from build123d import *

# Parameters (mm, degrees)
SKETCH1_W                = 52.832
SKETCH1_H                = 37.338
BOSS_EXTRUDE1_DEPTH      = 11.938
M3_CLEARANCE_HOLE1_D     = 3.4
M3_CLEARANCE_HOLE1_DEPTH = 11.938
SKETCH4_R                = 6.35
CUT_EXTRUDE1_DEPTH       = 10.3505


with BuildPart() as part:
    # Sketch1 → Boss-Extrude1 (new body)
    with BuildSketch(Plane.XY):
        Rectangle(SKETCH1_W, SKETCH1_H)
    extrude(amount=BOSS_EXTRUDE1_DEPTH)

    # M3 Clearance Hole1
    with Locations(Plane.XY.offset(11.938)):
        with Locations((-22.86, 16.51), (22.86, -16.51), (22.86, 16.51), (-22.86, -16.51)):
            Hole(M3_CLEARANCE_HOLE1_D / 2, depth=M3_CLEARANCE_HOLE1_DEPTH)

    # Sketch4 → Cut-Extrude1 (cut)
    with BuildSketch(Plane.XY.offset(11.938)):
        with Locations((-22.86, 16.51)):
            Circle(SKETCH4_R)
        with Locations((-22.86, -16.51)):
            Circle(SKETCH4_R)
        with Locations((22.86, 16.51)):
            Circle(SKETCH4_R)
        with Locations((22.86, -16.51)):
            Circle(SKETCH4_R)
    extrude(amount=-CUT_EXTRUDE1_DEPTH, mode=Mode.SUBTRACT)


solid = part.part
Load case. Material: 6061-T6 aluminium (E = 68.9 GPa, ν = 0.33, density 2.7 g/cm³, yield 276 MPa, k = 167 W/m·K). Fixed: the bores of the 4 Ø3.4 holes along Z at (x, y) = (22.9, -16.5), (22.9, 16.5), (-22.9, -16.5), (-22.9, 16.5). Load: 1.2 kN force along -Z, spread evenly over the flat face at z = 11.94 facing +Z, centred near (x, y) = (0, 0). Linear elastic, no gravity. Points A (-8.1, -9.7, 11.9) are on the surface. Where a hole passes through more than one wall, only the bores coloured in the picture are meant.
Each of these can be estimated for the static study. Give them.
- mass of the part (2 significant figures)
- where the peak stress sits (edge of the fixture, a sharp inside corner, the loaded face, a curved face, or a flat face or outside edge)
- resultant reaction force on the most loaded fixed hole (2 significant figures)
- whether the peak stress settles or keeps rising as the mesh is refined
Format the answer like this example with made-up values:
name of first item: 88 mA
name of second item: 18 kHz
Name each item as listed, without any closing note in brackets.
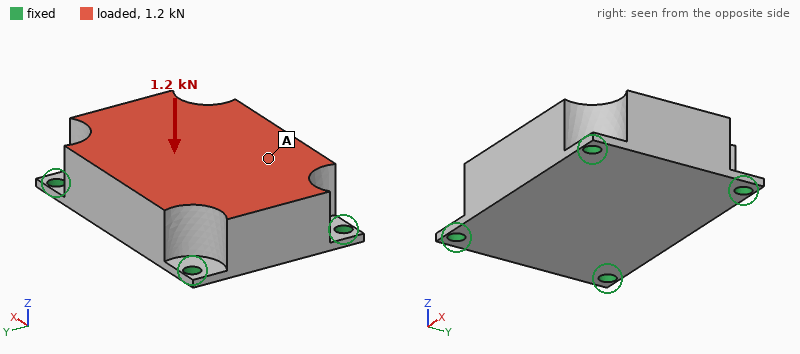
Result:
mass of the part: 55 g
where the peak stress sits: edge of the fixture
resultant reaction force on the most loaded fixed hole: 340 N
whether the peak stress settles or keeps rising as the mesh is refined: keeps rising
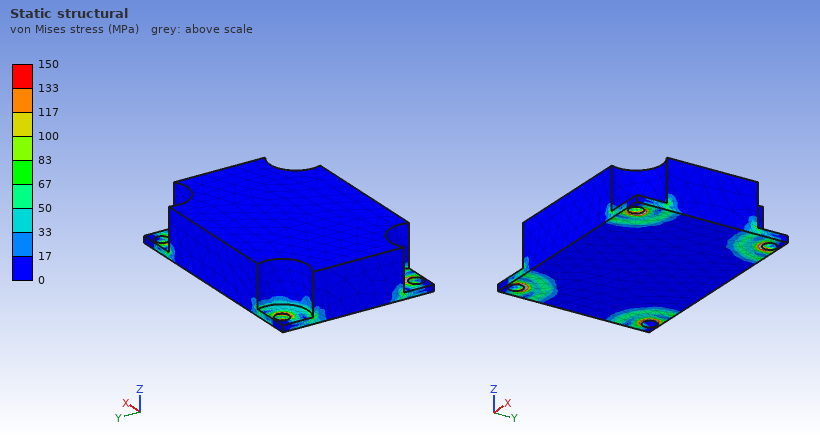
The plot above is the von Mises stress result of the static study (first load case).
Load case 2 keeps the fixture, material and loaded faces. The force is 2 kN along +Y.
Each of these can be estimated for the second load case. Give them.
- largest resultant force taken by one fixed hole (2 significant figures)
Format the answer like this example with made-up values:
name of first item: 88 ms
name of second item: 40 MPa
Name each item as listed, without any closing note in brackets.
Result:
largest resultant force taken by one fixed hole: 670 N
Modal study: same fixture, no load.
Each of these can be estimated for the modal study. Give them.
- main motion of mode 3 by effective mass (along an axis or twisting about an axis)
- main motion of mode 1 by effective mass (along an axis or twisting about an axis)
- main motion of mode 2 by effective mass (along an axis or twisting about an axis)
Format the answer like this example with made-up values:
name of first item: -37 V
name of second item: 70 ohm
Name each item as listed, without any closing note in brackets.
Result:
main motion of mode 3 by effective mass: along X
main motion of mode 1 by effective mass: along Z
main motion of mode 2 by effective mass: along Y
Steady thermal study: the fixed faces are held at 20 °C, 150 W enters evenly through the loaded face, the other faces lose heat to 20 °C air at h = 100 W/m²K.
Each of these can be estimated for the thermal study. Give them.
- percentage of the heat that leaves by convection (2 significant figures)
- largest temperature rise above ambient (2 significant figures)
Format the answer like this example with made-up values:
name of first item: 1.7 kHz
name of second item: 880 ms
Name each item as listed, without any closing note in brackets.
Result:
percentage of the heat that leaves by convection: 17 %
largest temperature rise above ambient: 73 K
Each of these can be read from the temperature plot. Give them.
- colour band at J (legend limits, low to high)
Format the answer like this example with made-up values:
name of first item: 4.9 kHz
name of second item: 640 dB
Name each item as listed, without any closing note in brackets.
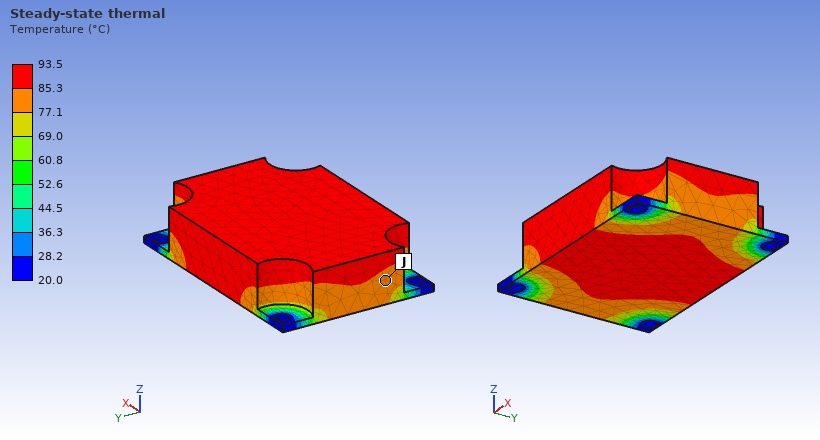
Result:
colour band at J: 77.1 to 85.3 °C
